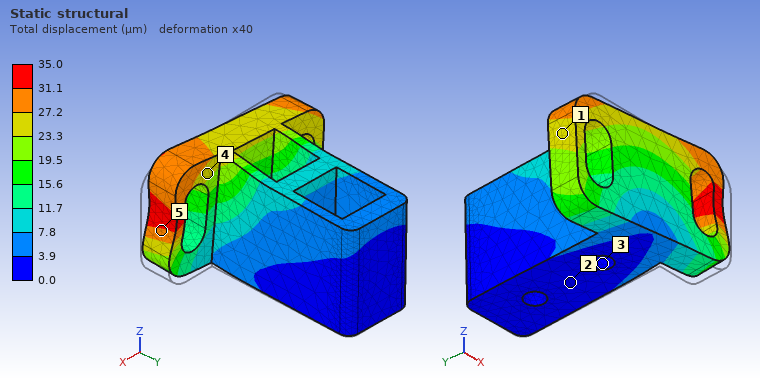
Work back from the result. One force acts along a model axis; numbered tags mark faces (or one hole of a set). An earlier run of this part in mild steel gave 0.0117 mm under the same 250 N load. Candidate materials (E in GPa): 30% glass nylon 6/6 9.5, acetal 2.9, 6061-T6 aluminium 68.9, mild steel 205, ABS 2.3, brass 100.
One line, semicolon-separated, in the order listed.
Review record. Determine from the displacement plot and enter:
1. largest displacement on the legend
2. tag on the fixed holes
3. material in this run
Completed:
35.0 µm; 3; 6061-T6 aluminium
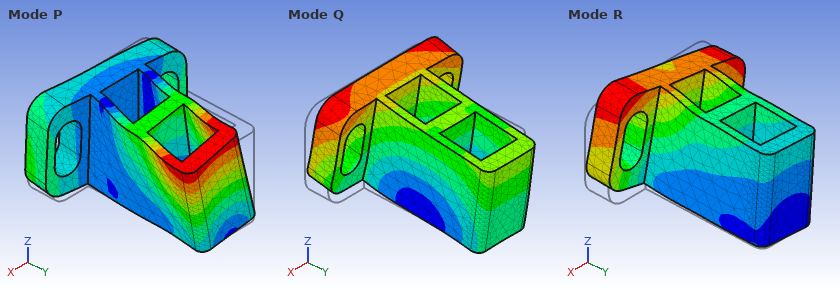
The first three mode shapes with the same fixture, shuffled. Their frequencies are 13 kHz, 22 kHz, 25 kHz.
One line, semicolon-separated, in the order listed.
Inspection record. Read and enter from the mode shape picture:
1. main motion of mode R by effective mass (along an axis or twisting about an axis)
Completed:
along X
